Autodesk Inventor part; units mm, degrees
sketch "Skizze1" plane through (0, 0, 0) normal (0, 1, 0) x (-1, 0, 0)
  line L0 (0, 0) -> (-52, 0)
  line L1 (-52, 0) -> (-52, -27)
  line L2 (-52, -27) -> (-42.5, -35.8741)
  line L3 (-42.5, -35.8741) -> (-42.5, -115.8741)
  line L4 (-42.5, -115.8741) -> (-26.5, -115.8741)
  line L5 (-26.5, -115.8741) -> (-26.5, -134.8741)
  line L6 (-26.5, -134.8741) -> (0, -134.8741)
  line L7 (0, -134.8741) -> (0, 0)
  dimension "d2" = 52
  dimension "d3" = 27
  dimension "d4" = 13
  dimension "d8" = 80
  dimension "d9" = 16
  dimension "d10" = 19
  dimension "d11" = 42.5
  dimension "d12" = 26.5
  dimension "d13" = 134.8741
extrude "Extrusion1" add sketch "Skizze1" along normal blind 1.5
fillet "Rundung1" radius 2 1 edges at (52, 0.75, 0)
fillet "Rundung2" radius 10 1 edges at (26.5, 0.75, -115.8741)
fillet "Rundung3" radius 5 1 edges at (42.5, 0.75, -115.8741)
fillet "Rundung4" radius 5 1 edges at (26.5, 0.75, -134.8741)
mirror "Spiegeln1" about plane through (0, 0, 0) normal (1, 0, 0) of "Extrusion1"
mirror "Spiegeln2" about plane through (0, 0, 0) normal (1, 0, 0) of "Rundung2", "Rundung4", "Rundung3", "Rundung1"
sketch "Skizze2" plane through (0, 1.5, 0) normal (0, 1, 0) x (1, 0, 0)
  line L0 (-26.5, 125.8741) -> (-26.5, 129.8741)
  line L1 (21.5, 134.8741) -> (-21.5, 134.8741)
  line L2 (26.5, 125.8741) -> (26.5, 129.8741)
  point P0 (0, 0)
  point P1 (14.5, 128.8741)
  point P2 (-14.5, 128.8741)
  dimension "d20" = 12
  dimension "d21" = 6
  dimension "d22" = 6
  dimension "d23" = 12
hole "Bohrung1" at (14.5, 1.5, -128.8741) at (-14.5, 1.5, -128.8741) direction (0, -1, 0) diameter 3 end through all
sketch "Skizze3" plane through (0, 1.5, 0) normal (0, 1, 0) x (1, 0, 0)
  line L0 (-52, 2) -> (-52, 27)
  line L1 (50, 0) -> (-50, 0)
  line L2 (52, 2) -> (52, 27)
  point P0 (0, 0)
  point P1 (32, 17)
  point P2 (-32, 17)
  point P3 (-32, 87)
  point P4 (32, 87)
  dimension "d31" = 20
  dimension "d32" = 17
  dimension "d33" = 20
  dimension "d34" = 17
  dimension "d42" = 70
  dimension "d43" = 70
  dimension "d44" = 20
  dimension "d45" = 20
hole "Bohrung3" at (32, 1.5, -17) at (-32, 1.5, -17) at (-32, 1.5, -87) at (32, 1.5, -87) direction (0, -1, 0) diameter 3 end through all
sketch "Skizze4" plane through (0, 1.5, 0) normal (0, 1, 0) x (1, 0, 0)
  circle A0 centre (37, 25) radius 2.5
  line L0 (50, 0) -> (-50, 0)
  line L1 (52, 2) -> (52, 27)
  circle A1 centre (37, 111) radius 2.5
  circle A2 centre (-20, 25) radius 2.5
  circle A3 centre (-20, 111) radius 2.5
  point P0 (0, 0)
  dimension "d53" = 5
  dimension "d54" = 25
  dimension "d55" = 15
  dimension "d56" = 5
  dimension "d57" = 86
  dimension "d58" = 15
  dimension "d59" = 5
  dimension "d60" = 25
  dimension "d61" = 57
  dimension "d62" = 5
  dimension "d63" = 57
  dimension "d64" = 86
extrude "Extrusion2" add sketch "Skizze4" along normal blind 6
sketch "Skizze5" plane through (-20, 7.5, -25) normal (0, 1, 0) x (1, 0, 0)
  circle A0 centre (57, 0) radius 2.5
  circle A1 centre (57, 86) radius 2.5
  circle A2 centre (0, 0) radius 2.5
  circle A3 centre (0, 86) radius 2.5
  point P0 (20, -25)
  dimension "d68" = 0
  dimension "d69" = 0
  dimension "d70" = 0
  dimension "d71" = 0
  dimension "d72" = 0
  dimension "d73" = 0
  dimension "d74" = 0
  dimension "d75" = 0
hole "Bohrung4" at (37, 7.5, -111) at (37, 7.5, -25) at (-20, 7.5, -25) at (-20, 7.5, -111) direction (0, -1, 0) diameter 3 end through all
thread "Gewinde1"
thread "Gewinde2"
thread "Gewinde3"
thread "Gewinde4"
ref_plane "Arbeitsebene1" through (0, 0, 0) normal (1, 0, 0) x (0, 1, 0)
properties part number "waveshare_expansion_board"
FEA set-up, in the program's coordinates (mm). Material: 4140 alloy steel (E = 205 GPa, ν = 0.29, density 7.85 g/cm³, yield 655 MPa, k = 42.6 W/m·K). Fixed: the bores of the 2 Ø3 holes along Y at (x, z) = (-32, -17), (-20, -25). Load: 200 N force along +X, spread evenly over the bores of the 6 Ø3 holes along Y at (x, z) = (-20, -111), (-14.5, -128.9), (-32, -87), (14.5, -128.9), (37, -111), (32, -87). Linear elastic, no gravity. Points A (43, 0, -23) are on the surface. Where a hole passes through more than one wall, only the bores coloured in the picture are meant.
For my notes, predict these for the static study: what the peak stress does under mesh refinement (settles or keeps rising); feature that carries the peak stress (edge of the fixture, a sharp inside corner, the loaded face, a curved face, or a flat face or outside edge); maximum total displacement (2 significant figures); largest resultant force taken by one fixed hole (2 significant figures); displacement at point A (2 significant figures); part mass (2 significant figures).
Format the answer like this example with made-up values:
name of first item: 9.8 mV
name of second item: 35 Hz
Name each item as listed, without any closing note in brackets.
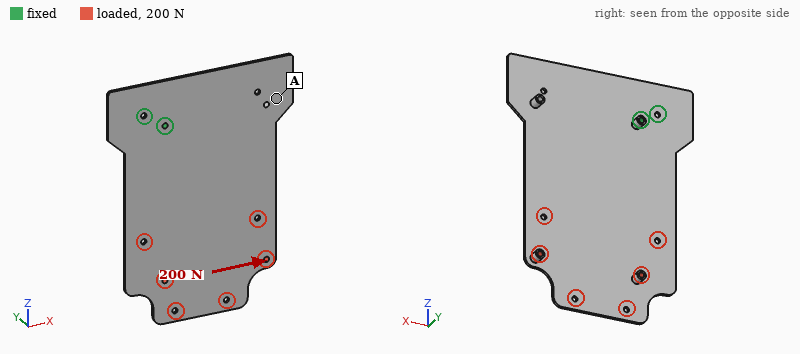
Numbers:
what the peak stress does under mesh refinement: keeps rising
feature that carries the peak stress: edge of the fixture
maximum total displacement: 0.32 mm
largest resultant force taken by one fixed hole: 1.1 kN
displacement at point A: 0.13 mm
part mass: 140 g
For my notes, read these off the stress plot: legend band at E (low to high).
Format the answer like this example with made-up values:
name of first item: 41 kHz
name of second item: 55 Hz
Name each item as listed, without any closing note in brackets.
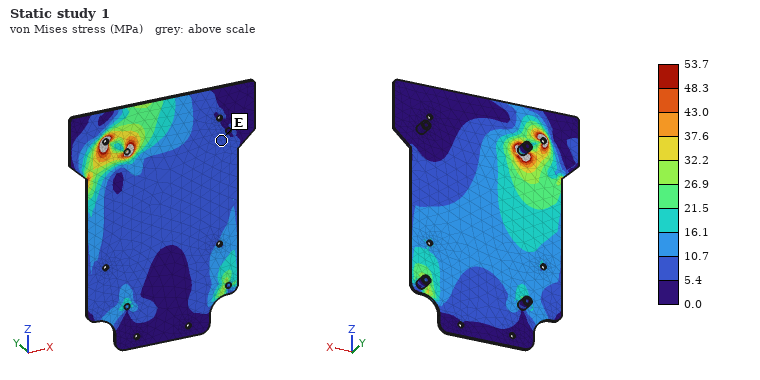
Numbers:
legend band at E: 5.4 to 10.7 MPa
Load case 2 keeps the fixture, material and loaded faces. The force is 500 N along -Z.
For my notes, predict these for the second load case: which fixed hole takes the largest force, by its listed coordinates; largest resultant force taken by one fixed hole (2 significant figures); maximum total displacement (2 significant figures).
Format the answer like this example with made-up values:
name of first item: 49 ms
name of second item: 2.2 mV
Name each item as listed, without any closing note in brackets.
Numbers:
which fixed hole takes the largest force, by its listed coordinates: (-20, -25)
largest resultant force taken by one fixed hole: 1.2 kN
maximum total displacement: 1.5 mm
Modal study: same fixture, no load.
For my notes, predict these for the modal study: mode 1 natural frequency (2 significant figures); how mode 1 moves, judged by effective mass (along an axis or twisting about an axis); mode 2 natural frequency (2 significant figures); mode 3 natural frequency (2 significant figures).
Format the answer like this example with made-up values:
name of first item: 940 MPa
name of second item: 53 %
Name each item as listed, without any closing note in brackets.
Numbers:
mode 1 natural frequency: 94 Hz
how mode 1 moves, judged by effective mass: along Y
mode 2 natural frequency: 210 Hz
mode 3 natural frequency: 410 Hz
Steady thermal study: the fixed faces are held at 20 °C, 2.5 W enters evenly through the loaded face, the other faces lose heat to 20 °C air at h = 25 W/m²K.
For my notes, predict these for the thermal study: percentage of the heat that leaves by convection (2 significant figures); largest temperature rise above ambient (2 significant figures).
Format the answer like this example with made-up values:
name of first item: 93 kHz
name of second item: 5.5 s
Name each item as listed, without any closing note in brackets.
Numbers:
percentage of the heat that leaves by convection: 94 %
largest temperature rise above ambient: 20 K
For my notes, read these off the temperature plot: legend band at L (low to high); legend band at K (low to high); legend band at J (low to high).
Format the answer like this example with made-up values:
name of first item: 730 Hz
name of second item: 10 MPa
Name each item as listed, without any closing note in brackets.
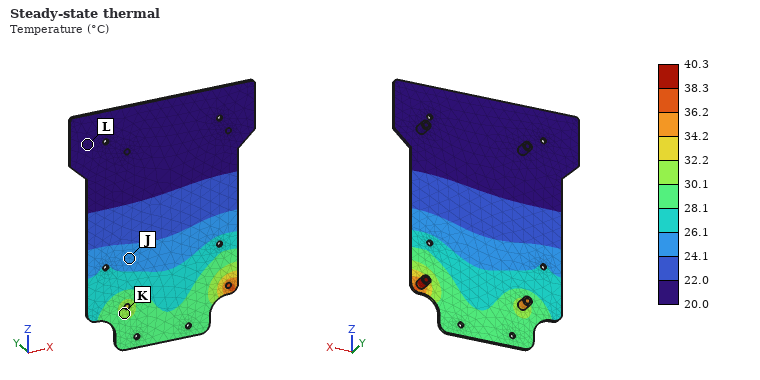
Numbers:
legend band at L: 20.0 to 22.0 °C
legend band at K: 30.1 to 32.2 °C
legend band at J: 24.1 to 26.1 °C
